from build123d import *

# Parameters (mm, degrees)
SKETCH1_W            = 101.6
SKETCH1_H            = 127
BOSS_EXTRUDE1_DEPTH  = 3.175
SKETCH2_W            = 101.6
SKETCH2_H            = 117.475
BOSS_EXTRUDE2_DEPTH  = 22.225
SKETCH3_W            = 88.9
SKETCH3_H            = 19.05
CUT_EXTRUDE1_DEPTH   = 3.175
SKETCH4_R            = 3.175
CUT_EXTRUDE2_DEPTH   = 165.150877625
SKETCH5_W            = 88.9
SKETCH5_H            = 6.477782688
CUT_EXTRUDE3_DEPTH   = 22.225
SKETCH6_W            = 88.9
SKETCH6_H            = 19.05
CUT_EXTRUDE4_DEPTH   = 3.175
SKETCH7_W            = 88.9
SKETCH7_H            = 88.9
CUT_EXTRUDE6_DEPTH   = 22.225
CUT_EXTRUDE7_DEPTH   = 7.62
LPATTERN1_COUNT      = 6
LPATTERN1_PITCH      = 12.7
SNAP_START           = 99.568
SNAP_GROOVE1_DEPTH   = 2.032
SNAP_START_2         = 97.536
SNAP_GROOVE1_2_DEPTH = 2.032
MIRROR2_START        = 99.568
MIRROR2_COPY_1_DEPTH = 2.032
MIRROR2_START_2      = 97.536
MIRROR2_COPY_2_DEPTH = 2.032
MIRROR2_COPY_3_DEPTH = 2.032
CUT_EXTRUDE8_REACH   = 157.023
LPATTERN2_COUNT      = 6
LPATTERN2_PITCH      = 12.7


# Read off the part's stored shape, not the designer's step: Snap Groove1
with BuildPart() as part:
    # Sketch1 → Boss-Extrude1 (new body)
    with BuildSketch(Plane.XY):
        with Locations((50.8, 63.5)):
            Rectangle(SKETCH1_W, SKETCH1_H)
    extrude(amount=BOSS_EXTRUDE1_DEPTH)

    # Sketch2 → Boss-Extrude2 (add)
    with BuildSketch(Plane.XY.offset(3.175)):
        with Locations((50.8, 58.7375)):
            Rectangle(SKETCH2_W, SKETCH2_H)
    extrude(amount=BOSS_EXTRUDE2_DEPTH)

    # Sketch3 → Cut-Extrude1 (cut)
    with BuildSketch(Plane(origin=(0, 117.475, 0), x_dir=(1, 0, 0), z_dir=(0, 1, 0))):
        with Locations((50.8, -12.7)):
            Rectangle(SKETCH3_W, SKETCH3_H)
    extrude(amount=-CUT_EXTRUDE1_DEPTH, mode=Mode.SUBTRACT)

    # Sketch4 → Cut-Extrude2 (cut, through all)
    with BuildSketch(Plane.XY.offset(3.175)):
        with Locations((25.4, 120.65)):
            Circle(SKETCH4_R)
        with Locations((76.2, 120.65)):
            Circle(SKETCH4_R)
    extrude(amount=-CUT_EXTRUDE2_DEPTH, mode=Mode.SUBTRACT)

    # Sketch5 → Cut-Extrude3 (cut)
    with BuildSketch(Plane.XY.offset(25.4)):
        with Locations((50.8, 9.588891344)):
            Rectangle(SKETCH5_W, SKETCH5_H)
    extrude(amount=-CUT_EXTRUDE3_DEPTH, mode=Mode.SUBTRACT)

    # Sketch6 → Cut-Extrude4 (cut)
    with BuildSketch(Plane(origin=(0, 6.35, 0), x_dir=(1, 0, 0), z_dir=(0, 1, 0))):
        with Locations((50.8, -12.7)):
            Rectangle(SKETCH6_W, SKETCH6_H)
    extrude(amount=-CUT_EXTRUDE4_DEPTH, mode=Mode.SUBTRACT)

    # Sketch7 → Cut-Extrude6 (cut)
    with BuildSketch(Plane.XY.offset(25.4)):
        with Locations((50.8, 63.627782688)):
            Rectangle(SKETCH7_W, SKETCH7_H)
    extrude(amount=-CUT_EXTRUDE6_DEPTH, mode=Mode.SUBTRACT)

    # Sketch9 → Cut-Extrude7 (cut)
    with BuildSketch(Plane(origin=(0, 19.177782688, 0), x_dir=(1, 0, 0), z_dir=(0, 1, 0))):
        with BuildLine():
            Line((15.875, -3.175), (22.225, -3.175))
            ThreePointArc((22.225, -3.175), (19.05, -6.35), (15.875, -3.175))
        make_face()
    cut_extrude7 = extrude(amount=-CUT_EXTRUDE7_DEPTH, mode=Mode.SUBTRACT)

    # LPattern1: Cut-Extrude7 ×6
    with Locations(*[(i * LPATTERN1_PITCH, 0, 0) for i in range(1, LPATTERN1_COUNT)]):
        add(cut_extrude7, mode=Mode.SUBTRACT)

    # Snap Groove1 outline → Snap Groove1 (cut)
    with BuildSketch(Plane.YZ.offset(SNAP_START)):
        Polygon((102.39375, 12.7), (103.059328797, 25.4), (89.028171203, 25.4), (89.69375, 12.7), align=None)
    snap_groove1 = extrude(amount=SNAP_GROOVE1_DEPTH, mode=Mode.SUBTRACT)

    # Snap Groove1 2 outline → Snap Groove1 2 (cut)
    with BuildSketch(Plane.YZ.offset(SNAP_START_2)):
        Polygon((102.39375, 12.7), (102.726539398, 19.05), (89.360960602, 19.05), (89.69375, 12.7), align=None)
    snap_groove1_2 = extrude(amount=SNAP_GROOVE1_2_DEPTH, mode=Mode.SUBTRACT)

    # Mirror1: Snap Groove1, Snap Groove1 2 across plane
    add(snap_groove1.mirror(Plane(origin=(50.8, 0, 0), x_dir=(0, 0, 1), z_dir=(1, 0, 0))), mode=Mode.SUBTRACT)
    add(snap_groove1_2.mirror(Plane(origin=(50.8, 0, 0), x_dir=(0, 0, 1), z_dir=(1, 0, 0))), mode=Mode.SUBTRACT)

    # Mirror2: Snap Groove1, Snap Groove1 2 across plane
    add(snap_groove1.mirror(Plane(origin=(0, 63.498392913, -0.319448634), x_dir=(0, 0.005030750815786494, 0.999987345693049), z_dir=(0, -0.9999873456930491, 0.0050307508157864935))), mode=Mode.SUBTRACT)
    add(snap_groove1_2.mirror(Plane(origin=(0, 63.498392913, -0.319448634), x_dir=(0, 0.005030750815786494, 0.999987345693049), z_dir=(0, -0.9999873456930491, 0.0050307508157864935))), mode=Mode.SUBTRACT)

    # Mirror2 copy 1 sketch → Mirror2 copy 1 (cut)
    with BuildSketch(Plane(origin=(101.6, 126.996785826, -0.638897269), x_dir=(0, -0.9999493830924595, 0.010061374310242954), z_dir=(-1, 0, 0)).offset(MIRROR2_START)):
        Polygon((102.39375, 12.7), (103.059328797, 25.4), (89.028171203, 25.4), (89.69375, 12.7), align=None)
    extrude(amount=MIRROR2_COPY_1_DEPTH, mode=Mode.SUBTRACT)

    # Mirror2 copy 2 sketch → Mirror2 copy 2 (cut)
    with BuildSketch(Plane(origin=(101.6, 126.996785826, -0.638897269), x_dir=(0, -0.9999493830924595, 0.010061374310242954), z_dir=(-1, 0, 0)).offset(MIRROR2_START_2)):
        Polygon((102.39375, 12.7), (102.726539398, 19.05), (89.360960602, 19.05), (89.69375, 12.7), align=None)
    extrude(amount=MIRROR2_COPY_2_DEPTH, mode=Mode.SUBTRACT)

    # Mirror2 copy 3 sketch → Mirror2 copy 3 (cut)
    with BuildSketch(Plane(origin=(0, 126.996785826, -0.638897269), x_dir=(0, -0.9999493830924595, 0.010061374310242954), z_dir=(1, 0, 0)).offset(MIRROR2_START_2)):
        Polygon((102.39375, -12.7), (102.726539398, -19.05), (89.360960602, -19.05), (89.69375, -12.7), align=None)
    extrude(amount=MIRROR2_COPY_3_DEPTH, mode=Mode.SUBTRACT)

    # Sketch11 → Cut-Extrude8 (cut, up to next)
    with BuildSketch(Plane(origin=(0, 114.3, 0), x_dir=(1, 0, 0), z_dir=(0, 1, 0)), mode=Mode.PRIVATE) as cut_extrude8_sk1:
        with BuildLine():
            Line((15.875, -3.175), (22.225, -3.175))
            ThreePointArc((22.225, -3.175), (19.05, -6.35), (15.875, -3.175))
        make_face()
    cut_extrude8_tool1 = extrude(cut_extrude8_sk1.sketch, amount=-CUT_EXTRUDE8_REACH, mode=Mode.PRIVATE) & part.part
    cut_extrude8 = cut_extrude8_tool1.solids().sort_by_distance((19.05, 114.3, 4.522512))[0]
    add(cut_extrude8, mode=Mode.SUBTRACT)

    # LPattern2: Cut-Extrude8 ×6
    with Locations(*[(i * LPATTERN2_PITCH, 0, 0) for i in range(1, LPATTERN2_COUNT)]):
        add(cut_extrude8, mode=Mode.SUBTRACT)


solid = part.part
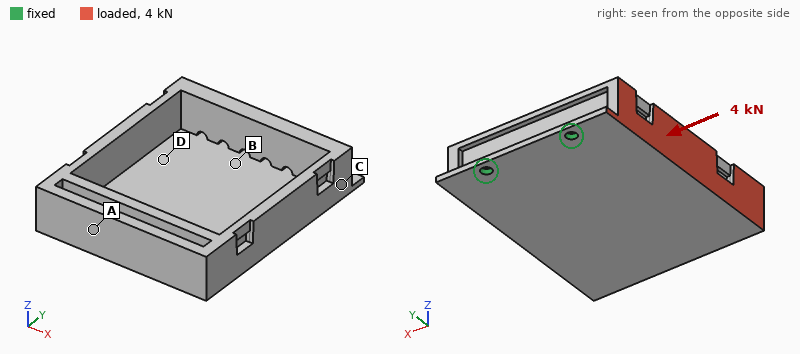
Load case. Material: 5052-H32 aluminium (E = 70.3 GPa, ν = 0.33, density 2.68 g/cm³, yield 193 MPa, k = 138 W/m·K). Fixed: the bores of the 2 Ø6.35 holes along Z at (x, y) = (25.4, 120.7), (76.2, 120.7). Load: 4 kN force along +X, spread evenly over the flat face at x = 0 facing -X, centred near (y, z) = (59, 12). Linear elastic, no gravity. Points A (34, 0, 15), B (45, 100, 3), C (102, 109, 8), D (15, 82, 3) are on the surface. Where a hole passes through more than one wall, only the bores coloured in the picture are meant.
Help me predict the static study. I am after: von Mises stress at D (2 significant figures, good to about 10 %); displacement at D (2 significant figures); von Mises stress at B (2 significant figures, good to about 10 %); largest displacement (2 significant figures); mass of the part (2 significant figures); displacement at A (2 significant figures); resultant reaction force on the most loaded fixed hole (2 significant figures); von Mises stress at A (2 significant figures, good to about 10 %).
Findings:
42 MPa
0.10 mm
49 MPa
0.58 mm
280 g
0.29 mm
5.0 kN
19 MPa
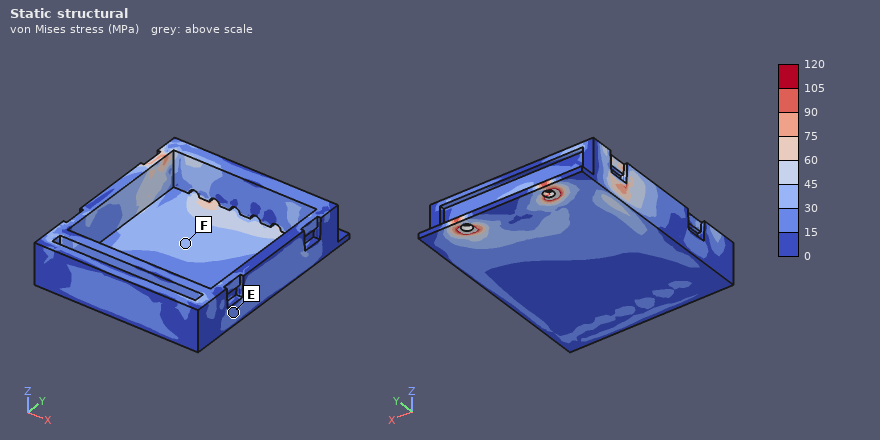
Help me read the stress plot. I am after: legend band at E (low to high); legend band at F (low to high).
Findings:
15 to 30 MPa
30 to 45 MPa
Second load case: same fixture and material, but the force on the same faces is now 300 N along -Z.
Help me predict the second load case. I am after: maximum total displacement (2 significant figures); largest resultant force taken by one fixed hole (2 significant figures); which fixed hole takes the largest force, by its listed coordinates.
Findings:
1.5 mm
440 N
(25.4, 120.7)
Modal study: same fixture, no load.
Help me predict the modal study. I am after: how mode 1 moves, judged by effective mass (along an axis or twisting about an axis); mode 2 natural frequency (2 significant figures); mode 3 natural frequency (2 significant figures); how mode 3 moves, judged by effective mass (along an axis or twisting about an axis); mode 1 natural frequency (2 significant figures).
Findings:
along Z
630 Hz
1700 Hz
along X
170 Hz
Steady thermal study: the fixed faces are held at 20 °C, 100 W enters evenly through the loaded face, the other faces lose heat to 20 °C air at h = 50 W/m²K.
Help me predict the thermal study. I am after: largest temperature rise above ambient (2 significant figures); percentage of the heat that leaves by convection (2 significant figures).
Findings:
64 K
63 %
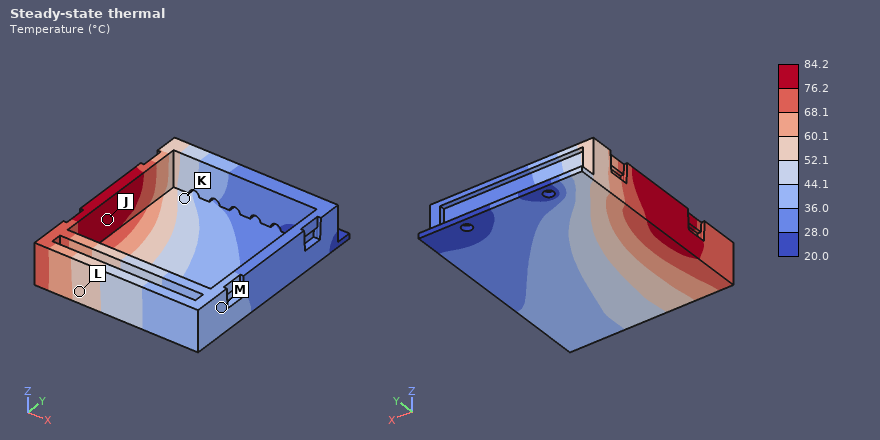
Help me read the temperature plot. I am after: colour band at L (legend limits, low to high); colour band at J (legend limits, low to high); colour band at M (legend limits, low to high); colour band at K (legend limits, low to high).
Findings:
52.1 to 60.1 °C
76.2 to 84.2 °C
36.0 to 44.1 °C
44.1 to 52.1 °C
